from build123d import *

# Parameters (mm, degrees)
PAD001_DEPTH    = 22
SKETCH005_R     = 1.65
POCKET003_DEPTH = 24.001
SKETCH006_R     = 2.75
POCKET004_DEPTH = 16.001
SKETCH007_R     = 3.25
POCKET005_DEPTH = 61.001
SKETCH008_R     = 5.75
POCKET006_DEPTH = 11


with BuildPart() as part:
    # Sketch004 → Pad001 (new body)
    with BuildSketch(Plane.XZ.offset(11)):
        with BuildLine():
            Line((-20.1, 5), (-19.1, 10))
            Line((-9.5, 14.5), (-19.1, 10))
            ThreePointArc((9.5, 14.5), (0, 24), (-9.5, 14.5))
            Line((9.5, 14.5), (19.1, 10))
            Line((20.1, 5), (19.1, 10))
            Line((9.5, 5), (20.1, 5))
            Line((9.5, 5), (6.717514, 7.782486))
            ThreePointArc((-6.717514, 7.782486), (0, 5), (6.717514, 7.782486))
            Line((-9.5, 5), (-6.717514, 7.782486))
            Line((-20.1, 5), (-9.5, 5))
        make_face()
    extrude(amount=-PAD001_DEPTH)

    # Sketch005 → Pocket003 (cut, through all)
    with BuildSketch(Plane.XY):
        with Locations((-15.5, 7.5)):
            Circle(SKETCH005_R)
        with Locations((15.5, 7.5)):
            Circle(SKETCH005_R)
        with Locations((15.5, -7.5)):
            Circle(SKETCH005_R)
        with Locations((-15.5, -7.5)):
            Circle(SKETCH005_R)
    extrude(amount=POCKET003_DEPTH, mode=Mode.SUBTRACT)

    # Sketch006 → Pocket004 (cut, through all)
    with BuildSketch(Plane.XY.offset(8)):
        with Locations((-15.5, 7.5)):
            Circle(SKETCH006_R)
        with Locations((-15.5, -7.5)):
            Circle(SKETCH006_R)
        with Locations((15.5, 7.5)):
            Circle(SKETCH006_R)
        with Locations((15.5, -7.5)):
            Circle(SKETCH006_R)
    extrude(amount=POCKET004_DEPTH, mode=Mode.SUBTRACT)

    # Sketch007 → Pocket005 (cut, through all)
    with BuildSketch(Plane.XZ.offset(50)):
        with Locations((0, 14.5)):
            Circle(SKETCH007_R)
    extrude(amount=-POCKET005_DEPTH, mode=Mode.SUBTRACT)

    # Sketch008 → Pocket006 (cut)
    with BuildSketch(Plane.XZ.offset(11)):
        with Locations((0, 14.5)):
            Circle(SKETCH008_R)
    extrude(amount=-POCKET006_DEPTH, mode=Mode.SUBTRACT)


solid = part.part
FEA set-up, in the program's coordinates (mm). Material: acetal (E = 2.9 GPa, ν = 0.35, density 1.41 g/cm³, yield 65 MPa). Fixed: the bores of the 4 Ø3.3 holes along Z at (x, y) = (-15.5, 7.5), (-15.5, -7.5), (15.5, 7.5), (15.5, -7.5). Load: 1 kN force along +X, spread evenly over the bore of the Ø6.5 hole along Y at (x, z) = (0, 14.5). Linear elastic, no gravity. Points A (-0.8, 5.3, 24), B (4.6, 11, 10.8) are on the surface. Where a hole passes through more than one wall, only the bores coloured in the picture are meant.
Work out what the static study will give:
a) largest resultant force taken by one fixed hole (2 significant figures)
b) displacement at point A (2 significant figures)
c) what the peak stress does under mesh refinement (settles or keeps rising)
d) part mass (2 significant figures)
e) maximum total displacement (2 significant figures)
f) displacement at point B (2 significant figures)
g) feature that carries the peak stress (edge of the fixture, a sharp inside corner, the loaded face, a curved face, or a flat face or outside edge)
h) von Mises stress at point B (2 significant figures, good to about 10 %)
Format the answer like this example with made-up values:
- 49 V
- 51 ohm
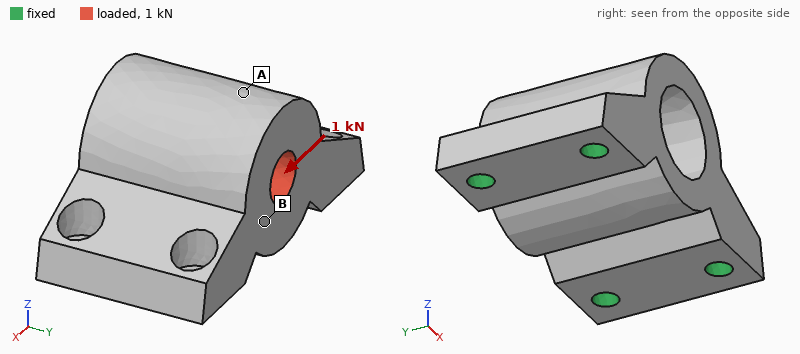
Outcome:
- 350 N
- 51 µm
- keeps rising
- 11 g
- 71 µm
- 38 µm
- edge of the fixture
- 5.9 MPa
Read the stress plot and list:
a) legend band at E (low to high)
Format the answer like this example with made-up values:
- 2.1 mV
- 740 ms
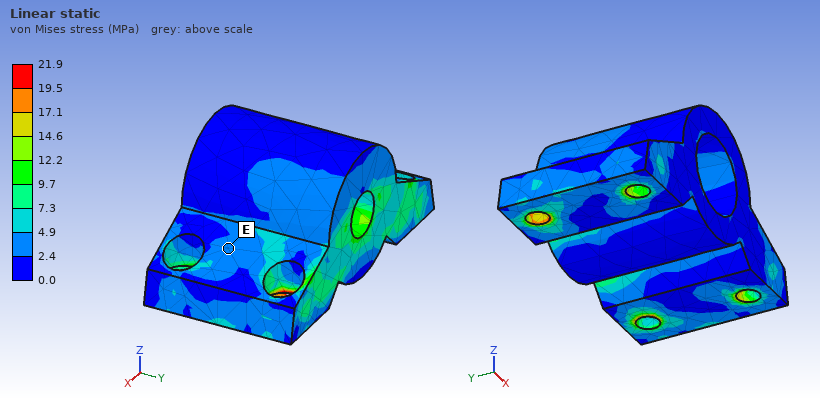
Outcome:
- 2.4 to 4.9 MPa
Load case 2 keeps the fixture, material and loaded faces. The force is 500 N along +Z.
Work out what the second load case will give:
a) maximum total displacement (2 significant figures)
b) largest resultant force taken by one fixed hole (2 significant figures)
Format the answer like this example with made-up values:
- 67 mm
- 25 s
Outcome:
- 76 µm
- 260 N
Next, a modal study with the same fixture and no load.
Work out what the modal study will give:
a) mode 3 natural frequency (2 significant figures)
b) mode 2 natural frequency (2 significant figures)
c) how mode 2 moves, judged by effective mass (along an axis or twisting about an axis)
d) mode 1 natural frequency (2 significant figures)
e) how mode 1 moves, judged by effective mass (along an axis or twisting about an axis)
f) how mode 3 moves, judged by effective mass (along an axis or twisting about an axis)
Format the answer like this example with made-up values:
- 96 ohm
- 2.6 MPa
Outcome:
- 8200 Hz
- 6600 Hz
- along Z
- 5300 Hz
- along Y
- along X
